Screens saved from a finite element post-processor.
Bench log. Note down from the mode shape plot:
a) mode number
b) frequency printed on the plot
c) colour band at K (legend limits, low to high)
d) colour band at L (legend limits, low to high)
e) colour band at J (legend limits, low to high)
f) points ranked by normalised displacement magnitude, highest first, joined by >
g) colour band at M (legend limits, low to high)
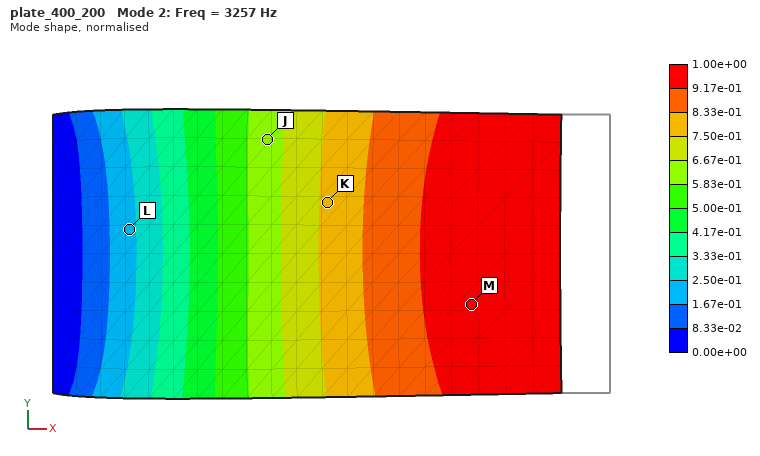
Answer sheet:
2
3257 Hz
7.50e-01 to 8.33e-01
1.67e-01 to 2.50e-01
5.83e-01 to 6.67e-01
M > K > J > L
9.17e-01 to 1.00e+00
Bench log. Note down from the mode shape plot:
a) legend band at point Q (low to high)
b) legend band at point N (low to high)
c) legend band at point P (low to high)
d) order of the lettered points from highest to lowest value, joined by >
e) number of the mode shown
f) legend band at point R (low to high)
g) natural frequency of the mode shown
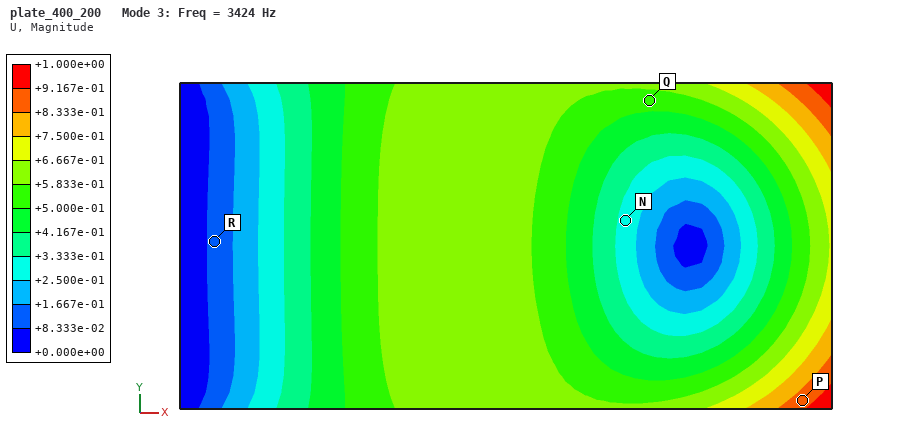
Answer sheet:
+5.000e-01 to +5.833e-01
+2.500e-01 to +3.333e-01
+8.333e-01 to +9.167e-01
P > Q > N > R
3
+8.333e-02 to +1.667e-01
3424 Hz
